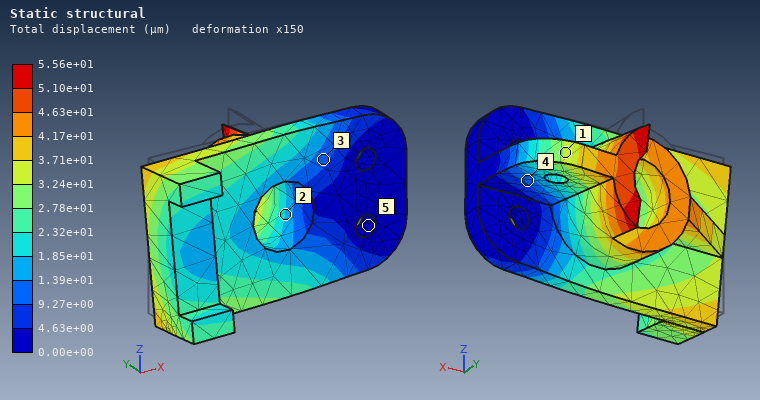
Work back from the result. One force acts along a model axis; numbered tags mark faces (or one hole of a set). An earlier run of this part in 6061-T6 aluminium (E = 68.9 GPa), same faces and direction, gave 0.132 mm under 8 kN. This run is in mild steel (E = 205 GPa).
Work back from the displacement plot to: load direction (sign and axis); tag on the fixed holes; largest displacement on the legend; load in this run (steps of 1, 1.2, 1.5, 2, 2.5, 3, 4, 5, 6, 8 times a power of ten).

-Z
5
5.56e+01 µm
10 kN
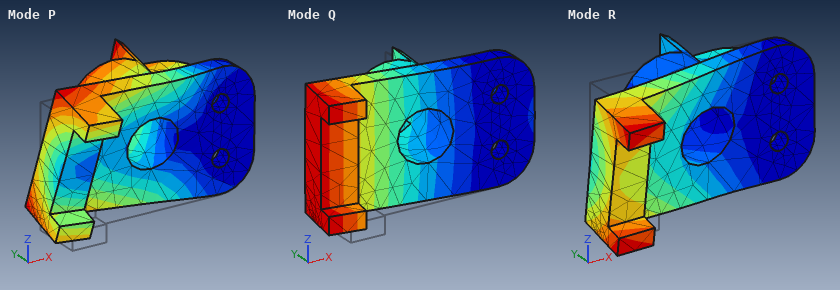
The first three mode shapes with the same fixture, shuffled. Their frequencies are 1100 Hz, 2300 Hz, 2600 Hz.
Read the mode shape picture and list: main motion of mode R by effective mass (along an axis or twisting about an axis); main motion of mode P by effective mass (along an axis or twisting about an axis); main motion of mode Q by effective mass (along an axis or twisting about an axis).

along Z
along Z
along Y
